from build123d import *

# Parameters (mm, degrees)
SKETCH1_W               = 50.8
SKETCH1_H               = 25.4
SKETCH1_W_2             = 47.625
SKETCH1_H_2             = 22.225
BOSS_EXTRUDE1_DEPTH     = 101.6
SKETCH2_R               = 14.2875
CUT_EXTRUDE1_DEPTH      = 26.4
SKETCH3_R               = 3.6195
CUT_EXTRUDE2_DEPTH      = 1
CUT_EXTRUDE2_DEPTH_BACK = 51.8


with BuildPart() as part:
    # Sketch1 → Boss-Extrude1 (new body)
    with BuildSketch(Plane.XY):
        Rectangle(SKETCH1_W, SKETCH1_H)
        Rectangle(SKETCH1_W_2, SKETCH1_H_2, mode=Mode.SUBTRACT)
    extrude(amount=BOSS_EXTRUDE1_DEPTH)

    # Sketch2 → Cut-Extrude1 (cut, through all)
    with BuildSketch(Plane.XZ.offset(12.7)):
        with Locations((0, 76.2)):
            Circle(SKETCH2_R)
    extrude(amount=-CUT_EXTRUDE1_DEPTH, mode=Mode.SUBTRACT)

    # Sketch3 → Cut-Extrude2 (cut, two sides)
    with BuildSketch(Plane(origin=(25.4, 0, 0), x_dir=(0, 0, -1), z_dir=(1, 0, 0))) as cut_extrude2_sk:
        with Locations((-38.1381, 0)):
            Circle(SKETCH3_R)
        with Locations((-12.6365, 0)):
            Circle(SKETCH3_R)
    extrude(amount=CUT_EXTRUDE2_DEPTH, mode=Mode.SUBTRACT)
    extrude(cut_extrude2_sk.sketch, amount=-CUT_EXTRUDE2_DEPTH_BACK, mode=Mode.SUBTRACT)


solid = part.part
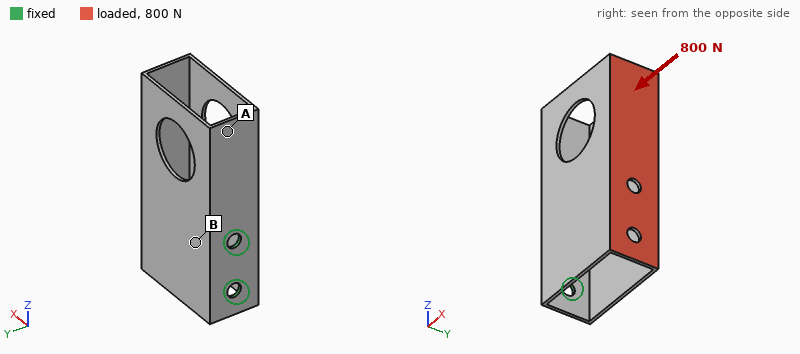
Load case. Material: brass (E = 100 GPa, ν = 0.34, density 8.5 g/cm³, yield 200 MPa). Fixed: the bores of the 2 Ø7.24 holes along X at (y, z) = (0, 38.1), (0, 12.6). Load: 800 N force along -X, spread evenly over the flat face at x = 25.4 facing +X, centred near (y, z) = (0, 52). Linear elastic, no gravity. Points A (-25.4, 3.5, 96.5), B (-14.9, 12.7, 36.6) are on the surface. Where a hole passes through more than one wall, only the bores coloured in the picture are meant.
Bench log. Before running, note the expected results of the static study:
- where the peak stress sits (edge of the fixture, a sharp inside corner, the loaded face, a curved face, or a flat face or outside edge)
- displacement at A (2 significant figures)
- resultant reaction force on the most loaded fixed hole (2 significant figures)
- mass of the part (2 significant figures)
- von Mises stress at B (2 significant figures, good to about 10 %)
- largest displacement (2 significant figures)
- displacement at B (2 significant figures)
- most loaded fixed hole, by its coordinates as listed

a flat face or outside edge
0.37 mm
1.1 kN
180 g
39 MPa
0.49 mm
0.12 mm
(0, 38.1)
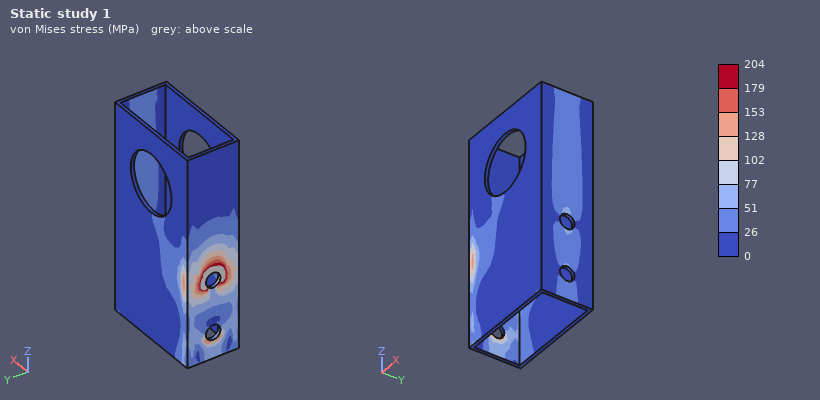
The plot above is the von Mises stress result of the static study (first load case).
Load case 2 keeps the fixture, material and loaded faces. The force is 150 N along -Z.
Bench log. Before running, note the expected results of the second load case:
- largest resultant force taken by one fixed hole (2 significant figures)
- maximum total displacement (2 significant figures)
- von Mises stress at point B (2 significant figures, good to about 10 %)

250 N
0.16 mm
8.5 MPa
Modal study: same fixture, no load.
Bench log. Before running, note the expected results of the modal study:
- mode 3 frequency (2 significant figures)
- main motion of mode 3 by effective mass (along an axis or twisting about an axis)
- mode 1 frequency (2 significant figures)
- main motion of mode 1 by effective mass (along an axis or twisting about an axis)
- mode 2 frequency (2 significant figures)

790 Hz
twisting about X
270 Hz
along Y
500 Hz
